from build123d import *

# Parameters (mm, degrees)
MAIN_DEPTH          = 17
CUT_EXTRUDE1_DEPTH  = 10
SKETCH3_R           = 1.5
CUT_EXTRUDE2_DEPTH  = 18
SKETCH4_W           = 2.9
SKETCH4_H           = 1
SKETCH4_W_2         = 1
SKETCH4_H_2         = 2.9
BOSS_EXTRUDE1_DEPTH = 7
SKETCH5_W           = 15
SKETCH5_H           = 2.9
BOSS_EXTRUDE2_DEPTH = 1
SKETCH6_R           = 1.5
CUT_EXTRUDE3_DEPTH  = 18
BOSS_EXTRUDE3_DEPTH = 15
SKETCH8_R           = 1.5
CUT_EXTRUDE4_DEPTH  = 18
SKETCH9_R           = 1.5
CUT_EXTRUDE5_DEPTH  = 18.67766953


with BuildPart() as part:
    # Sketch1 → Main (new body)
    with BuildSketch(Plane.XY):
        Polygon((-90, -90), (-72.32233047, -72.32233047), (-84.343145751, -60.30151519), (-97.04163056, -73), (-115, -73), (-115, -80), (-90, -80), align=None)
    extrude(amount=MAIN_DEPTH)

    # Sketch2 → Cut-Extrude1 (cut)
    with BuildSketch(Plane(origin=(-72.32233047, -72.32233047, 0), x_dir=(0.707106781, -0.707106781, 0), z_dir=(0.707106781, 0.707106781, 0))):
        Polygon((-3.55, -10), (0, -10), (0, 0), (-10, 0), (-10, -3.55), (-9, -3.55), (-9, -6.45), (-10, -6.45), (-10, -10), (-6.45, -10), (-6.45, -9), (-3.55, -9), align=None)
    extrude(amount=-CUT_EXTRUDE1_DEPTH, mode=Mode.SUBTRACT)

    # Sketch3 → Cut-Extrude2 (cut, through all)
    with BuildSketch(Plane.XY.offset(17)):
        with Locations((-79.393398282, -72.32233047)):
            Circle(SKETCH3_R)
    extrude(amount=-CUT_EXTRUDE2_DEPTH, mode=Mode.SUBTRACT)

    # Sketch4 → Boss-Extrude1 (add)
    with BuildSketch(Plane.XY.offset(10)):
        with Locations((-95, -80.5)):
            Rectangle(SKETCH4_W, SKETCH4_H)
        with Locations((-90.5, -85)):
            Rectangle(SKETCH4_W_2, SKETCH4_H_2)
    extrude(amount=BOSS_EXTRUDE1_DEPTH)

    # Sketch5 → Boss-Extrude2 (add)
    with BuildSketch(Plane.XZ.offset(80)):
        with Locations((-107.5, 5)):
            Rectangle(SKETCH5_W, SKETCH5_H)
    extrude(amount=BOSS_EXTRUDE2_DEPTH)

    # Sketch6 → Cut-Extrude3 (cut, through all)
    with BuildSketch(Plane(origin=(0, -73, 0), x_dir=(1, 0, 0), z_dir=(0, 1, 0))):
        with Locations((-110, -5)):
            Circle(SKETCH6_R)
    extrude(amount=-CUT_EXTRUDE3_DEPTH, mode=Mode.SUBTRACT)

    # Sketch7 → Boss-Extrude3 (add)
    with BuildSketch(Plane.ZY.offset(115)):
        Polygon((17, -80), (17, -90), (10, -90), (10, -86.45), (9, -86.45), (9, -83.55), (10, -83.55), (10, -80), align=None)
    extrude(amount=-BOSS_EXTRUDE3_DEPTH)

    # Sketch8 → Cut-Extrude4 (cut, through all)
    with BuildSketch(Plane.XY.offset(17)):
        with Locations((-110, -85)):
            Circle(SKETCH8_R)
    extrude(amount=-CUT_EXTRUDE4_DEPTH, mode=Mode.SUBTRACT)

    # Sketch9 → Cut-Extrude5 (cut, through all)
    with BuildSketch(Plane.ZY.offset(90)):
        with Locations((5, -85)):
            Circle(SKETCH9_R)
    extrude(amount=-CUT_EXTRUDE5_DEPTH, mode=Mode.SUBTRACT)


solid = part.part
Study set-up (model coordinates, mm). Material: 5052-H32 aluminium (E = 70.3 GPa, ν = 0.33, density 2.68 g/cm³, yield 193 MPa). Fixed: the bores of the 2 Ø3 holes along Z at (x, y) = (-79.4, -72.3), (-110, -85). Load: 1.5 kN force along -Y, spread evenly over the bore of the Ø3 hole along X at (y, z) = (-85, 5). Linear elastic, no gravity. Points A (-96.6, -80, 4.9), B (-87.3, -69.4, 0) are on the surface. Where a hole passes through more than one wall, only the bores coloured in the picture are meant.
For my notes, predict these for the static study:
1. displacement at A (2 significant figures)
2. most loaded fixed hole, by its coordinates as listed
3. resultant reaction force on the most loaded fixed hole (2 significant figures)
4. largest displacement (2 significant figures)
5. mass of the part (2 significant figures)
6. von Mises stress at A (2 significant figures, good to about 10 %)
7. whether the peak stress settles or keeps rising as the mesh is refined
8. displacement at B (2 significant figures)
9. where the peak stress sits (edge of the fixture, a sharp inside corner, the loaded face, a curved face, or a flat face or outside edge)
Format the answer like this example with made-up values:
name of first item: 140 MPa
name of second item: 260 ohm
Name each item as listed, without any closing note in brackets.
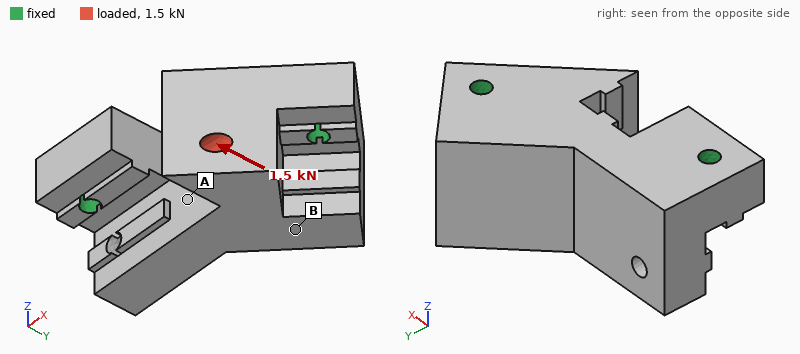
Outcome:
displacement at A: 17 µm
most loaded fixed hole, by its coordinates as listed: (-79.4, -72.3)
resultant reaction force on the most loaded fixed hole: 1.1 kN
largest displacement: 39 µm
mass of the part: 22 g
von Mises stress at A: 17 MPa
whether the peak stress settles or keeps rising as the mesh is refined: keeps rising
displacement at B: 27 µm
where the peak stress sits: edge of the fixture
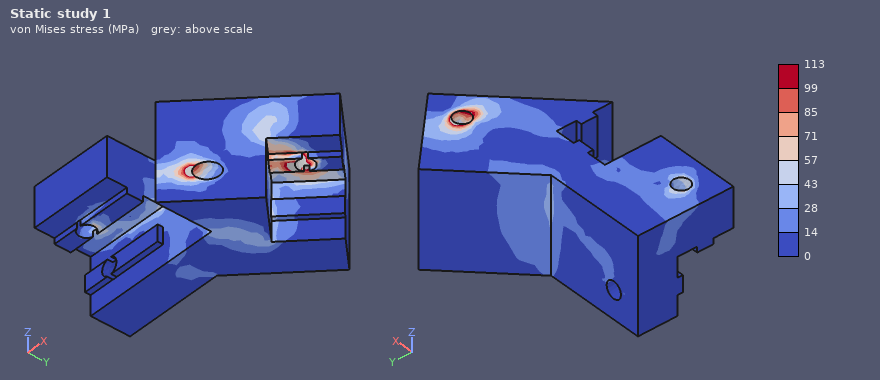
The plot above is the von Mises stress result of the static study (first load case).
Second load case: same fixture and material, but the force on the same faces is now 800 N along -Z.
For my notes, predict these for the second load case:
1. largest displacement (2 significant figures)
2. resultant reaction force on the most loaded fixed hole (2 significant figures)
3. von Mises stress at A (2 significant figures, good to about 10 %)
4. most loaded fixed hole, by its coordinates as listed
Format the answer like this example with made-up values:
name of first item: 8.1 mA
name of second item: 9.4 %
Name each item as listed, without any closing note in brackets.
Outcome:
largest displacement: 29 µm
resultant reaction force on the most loaded fixed hole: 580 N
von Mises stress at A: 14 MPa
most loaded fixed hole, by its coordinates as listed: (-79.4, -72.3)
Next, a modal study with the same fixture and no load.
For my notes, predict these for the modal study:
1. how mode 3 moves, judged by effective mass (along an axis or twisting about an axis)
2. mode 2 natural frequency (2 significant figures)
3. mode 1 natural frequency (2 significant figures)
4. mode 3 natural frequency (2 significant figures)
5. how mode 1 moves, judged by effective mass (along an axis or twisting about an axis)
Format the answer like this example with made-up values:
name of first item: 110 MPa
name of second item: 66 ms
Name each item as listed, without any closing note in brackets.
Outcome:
how mode 3 moves, judged by effective mass: along Z
mode 2 natural frequency: 18 kHz
mode 1 natural frequency: 12 kHz
mode 3 natural frequency: 21 kHz
how mode 1 moves, judged by effective mass: along Y
